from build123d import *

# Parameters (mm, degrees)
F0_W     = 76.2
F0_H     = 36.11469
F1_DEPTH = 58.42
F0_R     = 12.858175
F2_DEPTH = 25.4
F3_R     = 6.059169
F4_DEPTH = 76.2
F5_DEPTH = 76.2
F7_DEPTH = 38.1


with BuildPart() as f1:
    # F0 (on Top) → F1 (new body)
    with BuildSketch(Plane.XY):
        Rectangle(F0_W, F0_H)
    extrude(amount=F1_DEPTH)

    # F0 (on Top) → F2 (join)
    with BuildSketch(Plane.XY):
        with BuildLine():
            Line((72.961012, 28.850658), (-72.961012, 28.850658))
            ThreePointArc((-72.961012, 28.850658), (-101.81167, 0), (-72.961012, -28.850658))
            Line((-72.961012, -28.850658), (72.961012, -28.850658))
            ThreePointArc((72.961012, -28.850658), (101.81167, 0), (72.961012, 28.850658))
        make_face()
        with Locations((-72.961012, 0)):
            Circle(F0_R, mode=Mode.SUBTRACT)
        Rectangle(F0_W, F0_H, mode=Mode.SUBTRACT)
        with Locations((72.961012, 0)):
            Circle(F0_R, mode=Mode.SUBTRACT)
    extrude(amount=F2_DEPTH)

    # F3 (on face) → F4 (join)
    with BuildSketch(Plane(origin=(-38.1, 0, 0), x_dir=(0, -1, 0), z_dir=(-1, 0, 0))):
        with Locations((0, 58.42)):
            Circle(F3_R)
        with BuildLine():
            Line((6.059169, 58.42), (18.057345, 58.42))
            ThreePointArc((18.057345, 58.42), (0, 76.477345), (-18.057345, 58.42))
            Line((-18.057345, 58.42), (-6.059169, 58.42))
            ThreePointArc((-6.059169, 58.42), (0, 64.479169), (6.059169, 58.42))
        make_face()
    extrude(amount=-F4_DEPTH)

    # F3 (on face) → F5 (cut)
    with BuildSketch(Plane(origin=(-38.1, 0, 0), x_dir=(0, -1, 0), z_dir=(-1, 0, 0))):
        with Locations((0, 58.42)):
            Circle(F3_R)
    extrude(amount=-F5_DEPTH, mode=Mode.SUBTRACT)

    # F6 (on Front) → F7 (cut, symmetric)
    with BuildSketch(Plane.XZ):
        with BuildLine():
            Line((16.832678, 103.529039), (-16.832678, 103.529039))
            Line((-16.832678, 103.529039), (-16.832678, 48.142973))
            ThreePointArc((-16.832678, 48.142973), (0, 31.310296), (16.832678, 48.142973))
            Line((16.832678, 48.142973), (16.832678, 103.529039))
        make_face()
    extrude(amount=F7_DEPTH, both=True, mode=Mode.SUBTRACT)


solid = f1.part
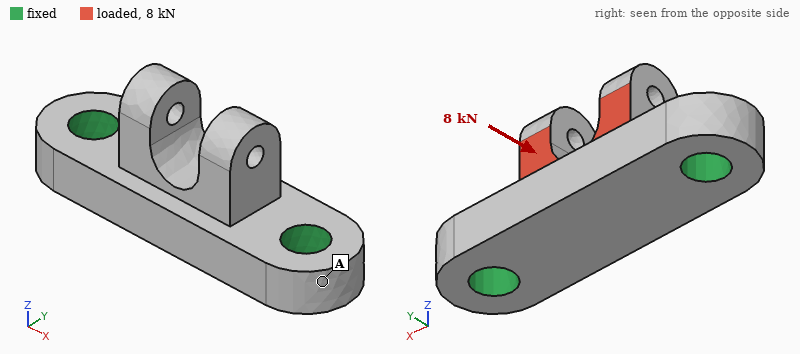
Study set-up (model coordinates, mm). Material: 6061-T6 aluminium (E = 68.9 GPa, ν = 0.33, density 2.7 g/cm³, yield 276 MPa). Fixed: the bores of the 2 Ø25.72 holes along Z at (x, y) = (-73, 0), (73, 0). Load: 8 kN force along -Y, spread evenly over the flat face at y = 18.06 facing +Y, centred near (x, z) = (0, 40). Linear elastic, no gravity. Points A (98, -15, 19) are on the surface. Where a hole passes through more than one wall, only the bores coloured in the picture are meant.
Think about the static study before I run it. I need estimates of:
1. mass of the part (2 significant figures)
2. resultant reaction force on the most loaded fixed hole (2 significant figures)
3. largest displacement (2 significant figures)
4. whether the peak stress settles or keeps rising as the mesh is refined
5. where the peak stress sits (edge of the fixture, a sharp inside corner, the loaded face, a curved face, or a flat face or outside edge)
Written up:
900 g
4.0 kN
50 µm
keeps rising
edge of the fixture
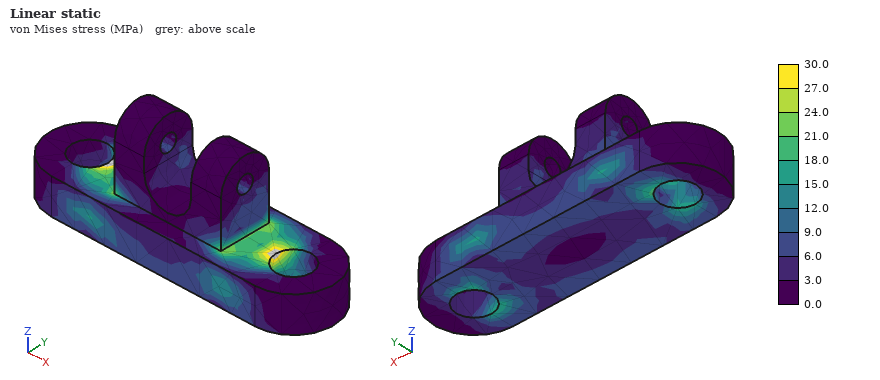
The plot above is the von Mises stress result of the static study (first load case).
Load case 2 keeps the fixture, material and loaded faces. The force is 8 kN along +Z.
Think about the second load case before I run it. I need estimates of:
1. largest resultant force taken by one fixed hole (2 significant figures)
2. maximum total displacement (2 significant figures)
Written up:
4.1 kN
35 µm
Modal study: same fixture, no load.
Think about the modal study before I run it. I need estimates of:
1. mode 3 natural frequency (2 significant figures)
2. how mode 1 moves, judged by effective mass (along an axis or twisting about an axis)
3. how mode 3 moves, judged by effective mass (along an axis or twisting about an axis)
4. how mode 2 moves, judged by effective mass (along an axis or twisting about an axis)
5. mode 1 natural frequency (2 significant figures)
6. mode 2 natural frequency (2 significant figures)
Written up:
7100 Hz
along Y
along X
along Z
4300 Hz
5300 Hz
